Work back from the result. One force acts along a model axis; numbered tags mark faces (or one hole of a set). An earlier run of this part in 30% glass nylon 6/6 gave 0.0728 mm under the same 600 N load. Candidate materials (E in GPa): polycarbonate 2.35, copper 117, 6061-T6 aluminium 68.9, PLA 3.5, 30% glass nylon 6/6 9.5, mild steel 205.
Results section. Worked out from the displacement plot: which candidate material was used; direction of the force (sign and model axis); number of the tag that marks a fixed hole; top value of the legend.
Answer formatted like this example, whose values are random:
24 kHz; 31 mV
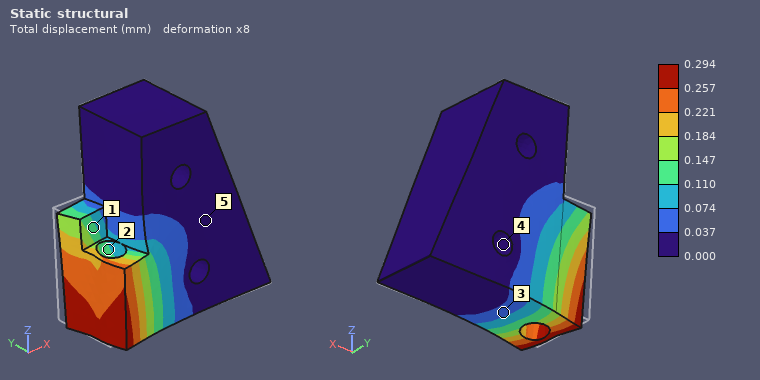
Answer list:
polycarbonate; -Y; 4; 0.294 mm
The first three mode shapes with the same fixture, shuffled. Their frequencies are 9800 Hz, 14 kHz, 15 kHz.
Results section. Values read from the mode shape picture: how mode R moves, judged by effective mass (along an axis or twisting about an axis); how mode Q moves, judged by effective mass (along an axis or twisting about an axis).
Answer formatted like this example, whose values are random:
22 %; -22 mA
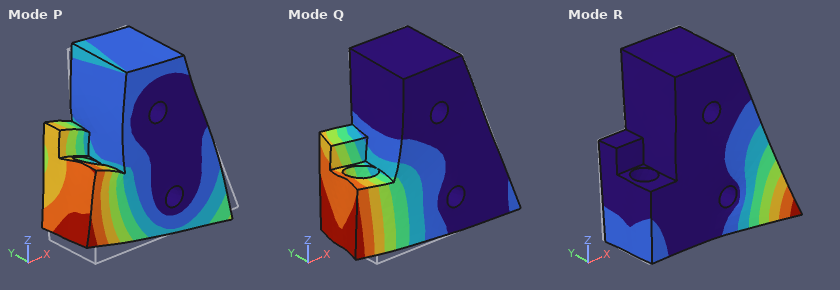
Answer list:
along Y; along Y
